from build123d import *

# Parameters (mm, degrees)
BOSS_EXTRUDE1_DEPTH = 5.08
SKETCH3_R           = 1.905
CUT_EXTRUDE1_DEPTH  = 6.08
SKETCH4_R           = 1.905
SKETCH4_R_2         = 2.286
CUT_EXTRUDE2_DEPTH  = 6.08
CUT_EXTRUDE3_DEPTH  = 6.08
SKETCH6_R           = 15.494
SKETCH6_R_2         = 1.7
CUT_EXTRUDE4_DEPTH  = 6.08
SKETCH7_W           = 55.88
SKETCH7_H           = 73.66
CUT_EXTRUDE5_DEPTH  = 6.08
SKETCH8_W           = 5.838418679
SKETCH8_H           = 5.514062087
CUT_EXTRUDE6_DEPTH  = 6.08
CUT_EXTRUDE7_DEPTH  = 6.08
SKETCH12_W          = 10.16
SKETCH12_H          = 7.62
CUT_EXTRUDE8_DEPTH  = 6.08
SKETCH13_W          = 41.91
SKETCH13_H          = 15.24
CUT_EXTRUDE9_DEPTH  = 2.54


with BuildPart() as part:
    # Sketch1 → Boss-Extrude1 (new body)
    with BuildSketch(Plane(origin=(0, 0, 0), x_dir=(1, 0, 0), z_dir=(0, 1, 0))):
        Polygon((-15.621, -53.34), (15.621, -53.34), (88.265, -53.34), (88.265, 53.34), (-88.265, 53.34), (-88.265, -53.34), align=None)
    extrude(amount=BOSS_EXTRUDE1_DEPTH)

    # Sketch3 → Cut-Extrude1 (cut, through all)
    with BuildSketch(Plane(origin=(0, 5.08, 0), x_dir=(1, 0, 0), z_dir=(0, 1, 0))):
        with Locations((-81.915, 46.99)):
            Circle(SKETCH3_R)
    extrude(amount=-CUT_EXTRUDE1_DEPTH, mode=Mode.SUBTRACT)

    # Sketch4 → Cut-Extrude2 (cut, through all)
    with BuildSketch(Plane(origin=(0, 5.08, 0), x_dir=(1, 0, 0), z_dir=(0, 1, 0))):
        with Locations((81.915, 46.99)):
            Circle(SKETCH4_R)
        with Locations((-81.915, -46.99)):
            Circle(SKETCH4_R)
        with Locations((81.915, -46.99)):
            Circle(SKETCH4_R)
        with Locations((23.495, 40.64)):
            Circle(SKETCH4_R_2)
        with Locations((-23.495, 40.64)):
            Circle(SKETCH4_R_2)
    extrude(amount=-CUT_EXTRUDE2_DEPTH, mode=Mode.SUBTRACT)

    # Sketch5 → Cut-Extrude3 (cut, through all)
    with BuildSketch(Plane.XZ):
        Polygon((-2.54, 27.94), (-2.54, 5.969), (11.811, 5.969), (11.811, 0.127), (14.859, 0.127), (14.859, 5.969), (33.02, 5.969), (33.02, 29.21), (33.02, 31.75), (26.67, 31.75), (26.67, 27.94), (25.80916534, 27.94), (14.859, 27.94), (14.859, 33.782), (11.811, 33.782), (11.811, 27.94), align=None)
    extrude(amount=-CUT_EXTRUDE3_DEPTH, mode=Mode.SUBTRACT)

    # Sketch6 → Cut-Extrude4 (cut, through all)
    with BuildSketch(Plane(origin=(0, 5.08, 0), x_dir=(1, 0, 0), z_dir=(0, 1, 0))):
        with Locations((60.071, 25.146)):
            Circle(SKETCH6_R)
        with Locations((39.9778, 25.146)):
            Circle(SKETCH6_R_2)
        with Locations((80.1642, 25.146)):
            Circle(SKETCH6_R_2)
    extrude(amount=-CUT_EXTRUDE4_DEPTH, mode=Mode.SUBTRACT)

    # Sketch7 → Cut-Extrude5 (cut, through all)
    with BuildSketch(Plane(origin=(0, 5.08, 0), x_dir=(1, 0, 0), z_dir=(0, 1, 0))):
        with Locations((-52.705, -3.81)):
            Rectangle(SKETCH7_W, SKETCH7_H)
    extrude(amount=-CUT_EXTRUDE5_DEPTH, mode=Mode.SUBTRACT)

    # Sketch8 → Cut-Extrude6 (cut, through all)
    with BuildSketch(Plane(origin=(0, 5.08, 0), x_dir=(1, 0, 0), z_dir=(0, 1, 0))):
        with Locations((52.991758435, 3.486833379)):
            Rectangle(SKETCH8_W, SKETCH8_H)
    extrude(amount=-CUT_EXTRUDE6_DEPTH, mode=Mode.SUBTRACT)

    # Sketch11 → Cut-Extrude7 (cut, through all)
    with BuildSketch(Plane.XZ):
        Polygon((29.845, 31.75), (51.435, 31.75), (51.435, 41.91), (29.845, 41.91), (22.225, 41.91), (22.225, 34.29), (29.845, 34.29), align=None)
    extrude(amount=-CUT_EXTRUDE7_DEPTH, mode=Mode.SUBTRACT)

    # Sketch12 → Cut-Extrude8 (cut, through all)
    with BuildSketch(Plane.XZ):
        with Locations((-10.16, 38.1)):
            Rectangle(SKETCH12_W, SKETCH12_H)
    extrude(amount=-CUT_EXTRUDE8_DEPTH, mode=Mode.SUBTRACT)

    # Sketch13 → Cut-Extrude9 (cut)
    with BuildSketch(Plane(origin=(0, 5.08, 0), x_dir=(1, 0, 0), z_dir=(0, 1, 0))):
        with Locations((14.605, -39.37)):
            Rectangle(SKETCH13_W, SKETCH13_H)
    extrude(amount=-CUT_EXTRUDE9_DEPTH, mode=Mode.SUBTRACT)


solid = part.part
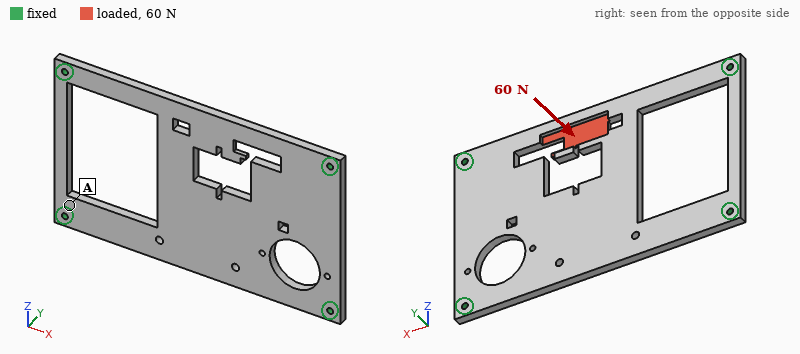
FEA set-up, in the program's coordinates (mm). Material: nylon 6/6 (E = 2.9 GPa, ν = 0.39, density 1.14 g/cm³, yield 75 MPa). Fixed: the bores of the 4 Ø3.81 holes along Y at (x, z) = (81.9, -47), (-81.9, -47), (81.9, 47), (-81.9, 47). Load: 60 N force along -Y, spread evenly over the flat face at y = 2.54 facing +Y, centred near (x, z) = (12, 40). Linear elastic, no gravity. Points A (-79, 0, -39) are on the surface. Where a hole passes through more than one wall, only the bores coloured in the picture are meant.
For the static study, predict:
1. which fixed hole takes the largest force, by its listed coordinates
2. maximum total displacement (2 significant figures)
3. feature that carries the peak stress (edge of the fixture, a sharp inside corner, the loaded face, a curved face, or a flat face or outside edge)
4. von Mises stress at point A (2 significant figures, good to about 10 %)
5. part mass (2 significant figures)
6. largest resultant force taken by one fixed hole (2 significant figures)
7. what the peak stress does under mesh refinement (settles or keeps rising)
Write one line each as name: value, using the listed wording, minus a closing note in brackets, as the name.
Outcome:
which fixed hole takes the largest force, by its listed coordinates: (81.9, 47)
maximum total displacement: 2.1 mm
feature that carries the peak stress: edge of the fixture
von Mises stress at point A: 2.0 MPa
part mass: 72 g
largest resultant force taken by one fixed hole: 45 N
what the peak stress does under mesh refinement: keeps rising
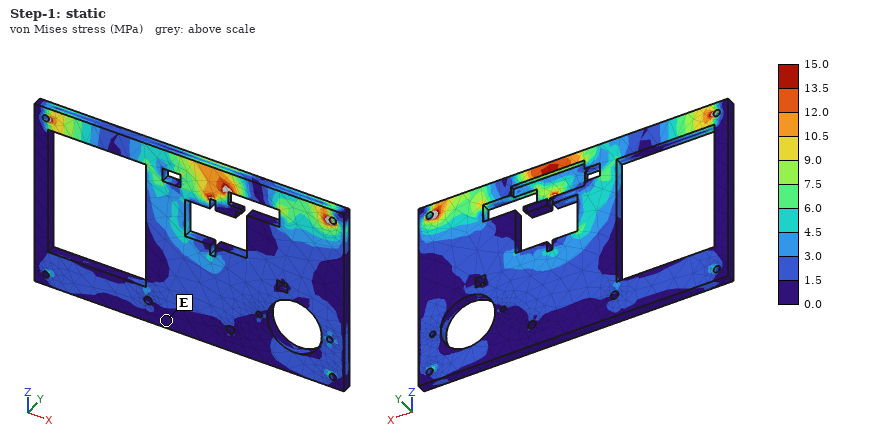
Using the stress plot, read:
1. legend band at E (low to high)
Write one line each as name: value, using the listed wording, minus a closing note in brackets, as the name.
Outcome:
legend band at E: 0.0 to 1.5 MPa
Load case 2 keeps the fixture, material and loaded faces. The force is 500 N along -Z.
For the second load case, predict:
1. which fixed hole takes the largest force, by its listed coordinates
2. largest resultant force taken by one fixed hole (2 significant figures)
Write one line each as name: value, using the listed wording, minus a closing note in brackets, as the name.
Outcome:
which fixed hole takes the largest force, by its listed coordinates: (81.9, 47)
largest resultant force taken by one fixed hole: 400 N
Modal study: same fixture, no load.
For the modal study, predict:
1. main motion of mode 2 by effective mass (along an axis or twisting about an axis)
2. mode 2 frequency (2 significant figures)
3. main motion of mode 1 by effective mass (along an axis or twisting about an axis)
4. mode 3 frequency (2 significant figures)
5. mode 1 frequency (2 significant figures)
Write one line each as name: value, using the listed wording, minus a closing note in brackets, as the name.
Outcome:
main motion of mode 2 by effective mass: twisting about X
mode 2 frequency: 360 Hz
main motion of mode 1 by effective mass: along Y
mode 3 frequency: 600 Hz
mode 1 frequency: 220 Hz
